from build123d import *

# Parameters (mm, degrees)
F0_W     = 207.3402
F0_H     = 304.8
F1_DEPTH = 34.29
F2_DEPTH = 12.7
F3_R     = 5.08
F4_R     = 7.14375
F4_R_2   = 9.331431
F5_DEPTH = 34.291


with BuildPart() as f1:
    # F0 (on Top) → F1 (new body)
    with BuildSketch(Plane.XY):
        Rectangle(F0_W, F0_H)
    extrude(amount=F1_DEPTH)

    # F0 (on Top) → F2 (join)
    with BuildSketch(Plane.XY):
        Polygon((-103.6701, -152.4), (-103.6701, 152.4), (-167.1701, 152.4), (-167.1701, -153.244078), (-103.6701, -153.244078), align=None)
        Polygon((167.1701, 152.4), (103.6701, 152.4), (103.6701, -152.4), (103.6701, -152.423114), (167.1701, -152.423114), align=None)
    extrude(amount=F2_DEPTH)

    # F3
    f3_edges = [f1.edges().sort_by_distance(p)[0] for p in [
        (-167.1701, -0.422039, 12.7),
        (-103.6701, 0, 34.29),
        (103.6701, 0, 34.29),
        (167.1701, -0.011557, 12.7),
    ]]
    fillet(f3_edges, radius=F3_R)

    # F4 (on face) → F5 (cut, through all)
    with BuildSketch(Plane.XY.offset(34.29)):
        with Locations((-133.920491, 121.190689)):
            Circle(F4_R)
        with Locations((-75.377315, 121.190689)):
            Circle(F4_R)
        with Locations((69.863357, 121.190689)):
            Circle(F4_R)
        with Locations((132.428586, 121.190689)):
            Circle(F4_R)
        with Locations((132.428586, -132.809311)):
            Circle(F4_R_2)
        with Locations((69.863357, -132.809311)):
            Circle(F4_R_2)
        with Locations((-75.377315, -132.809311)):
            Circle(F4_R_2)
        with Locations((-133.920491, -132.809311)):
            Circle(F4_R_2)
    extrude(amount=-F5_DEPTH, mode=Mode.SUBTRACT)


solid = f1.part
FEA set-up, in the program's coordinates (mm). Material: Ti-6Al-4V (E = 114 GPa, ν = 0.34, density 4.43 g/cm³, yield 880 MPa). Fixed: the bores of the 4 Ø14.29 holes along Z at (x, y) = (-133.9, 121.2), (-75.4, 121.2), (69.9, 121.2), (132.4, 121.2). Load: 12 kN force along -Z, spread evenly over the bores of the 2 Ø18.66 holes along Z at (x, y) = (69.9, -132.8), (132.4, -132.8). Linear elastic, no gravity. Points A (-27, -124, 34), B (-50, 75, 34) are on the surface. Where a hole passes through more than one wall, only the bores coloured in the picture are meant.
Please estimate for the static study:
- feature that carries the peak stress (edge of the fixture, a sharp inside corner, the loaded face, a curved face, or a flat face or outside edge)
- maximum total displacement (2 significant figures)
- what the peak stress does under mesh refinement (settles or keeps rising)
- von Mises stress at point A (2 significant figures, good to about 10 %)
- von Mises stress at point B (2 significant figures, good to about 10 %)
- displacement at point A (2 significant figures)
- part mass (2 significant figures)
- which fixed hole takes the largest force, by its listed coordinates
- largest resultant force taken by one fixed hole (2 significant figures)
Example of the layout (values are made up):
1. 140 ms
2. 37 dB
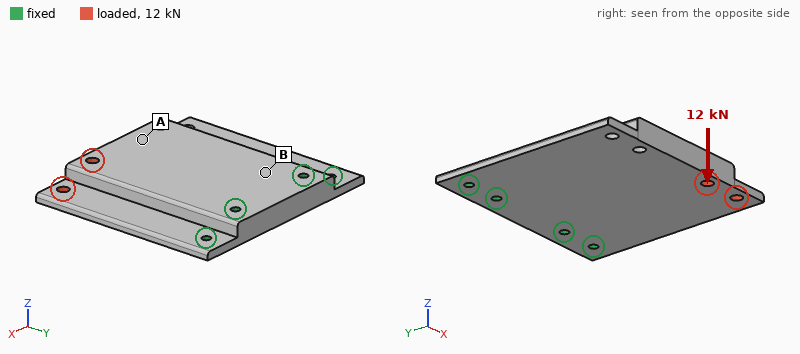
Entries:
1. edge of the fixture
2. 1.3 mm
3. keeps rising
4. 16 MPa
5. 48 MPa
6. 0.72 mm
7. 12 kg
8. (69.9, 121.2)
9. 27 kN
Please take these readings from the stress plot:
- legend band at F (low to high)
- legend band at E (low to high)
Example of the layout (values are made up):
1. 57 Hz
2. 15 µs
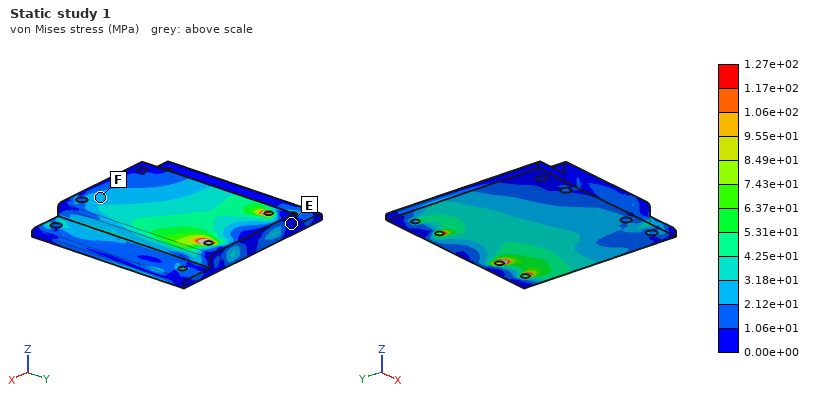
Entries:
1. 2.12e+01 to 3.18e+01 MPa
2. 0.00e+00 to 1.06e+01 MPa
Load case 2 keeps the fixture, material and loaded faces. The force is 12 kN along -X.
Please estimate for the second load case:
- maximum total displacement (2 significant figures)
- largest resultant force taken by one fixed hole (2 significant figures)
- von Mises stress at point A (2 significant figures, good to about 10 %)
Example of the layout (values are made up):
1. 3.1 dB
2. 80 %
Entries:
1. 44 µm
2. 9.8 kN
3. 1.4 MPa
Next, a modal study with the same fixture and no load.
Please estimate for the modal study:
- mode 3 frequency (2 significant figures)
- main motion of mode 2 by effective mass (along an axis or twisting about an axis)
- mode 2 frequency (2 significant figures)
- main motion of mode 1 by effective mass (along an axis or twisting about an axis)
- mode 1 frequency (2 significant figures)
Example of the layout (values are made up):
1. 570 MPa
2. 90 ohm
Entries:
1. 1700 Hz
2. twisting about Y
3. 750 Hz
4. along Z
5. 340 Hz
